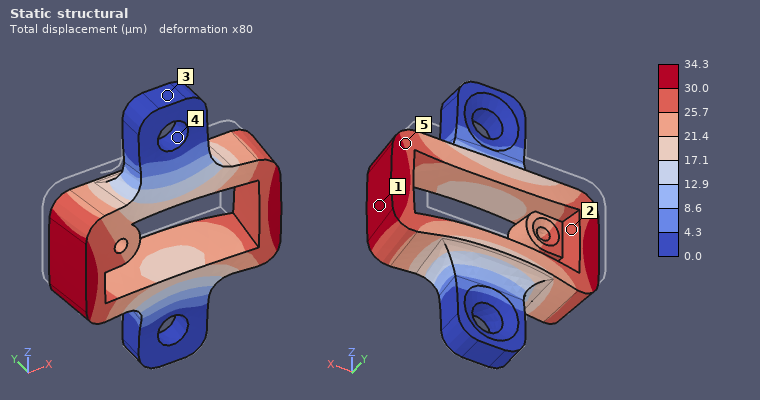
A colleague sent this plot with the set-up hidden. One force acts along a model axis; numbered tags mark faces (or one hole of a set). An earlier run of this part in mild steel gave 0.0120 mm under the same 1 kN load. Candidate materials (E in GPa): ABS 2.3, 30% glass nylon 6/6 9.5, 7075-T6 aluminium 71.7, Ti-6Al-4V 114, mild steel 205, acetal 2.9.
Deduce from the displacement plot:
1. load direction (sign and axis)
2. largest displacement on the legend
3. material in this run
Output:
-Y
34.3 µm
7075-T6 aluminium
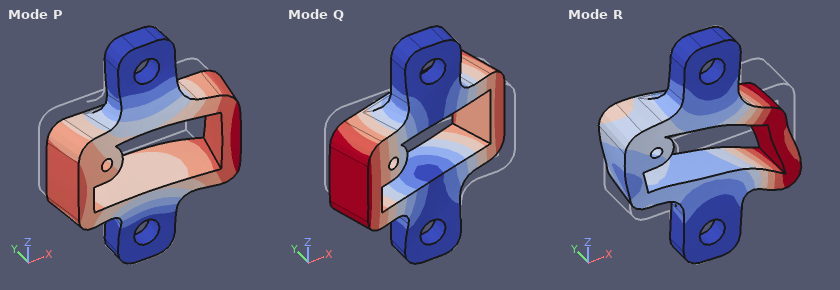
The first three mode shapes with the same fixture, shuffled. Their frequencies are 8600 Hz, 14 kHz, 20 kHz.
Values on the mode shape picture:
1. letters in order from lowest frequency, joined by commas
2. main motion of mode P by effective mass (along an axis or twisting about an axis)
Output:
Q, P, R
along Y
